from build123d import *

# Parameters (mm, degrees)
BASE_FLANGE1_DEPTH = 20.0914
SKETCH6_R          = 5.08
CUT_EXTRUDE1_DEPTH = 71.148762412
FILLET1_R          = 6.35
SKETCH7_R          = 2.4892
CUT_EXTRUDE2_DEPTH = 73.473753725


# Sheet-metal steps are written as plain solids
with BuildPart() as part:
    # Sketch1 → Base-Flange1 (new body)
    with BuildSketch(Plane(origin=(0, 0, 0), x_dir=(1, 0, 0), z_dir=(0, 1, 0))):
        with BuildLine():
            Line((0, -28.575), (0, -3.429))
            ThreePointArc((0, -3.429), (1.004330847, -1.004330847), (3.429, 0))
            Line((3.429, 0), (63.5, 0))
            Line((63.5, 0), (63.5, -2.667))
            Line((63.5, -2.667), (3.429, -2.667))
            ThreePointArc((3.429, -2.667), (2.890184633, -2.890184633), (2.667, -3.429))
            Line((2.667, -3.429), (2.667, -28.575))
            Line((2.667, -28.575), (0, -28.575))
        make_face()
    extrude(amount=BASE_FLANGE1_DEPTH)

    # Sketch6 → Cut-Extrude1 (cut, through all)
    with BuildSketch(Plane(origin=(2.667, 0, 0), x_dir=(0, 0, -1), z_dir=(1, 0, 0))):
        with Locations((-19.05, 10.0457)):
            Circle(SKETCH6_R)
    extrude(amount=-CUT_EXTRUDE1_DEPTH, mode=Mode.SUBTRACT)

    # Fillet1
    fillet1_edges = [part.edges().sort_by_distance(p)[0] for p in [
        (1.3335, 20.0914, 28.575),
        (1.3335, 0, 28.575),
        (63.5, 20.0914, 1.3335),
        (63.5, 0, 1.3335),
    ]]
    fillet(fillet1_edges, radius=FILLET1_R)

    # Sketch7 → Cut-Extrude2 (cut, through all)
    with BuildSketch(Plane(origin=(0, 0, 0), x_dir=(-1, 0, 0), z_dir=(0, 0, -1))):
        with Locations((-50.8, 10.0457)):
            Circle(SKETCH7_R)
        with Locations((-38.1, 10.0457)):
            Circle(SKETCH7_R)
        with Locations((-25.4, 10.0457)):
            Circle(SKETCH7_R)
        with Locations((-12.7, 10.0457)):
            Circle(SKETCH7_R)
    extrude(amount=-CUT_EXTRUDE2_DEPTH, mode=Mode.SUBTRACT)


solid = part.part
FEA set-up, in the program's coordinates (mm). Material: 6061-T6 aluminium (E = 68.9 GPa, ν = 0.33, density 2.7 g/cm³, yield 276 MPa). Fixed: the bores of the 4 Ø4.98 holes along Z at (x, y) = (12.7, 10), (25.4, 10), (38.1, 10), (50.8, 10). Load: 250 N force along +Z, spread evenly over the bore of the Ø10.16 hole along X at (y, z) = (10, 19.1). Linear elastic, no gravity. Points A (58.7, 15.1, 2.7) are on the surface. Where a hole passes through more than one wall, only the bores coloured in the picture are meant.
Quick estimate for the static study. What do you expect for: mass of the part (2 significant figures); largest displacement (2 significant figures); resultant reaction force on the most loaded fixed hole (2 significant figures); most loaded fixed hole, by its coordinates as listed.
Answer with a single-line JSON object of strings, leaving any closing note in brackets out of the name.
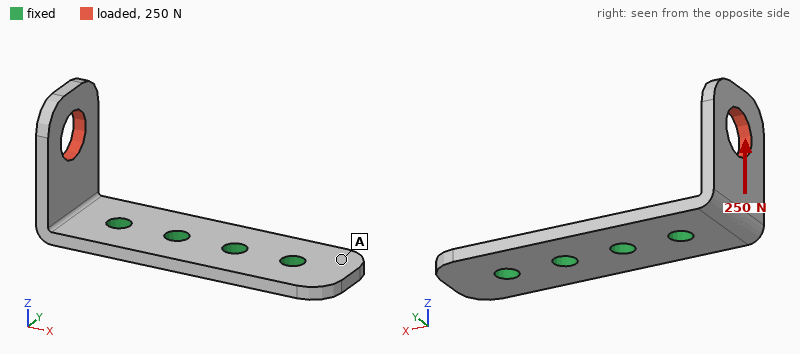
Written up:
{"mass of the part": "11 g", "largest displacement": "0.17 mm", "resultant reaction force on the most loaded fixed hole": "290 N", "most loaded fixed hole, by its coordinates as listed": "(12.7, 10)"}
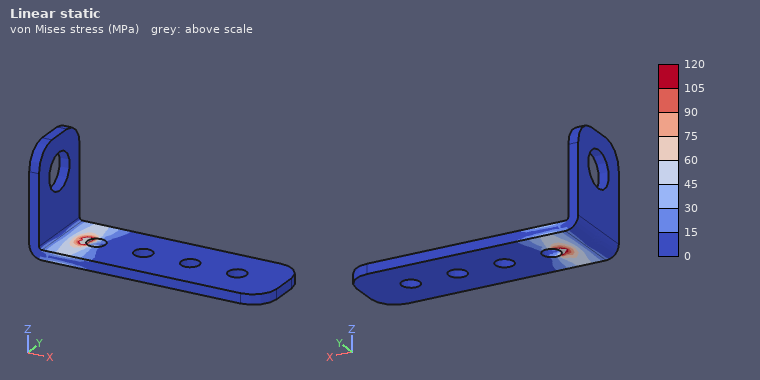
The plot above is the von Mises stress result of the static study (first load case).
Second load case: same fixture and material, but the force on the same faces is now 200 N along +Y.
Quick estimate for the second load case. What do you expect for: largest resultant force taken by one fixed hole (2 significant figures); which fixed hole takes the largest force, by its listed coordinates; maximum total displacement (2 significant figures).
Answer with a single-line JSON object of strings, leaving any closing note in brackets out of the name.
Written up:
{"largest resultant force taken by one fixed hole": "280 N", "which fixed hole takes the largest force, by its listed coordinates": "(12.7, 10)", "maximum total displacement": "0.25 mm"}
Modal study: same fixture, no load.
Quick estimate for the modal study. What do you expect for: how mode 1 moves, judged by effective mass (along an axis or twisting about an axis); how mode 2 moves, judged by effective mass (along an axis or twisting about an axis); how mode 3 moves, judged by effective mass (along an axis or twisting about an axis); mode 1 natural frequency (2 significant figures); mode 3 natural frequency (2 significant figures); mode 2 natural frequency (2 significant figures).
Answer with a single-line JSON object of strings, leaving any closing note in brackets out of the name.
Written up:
{"how mode 1 moves, judged by effective mass": "along X", "how mode 2 moves, judged by effective mass": "along Y", "how mode 3 moves, judged by effective mass": "along Z", "mode 1 natural frequency": "2200 Hz", "mode 3 natural frequency": "8100 Hz", "mode 2 natural frequency": "3400 Hz"}
